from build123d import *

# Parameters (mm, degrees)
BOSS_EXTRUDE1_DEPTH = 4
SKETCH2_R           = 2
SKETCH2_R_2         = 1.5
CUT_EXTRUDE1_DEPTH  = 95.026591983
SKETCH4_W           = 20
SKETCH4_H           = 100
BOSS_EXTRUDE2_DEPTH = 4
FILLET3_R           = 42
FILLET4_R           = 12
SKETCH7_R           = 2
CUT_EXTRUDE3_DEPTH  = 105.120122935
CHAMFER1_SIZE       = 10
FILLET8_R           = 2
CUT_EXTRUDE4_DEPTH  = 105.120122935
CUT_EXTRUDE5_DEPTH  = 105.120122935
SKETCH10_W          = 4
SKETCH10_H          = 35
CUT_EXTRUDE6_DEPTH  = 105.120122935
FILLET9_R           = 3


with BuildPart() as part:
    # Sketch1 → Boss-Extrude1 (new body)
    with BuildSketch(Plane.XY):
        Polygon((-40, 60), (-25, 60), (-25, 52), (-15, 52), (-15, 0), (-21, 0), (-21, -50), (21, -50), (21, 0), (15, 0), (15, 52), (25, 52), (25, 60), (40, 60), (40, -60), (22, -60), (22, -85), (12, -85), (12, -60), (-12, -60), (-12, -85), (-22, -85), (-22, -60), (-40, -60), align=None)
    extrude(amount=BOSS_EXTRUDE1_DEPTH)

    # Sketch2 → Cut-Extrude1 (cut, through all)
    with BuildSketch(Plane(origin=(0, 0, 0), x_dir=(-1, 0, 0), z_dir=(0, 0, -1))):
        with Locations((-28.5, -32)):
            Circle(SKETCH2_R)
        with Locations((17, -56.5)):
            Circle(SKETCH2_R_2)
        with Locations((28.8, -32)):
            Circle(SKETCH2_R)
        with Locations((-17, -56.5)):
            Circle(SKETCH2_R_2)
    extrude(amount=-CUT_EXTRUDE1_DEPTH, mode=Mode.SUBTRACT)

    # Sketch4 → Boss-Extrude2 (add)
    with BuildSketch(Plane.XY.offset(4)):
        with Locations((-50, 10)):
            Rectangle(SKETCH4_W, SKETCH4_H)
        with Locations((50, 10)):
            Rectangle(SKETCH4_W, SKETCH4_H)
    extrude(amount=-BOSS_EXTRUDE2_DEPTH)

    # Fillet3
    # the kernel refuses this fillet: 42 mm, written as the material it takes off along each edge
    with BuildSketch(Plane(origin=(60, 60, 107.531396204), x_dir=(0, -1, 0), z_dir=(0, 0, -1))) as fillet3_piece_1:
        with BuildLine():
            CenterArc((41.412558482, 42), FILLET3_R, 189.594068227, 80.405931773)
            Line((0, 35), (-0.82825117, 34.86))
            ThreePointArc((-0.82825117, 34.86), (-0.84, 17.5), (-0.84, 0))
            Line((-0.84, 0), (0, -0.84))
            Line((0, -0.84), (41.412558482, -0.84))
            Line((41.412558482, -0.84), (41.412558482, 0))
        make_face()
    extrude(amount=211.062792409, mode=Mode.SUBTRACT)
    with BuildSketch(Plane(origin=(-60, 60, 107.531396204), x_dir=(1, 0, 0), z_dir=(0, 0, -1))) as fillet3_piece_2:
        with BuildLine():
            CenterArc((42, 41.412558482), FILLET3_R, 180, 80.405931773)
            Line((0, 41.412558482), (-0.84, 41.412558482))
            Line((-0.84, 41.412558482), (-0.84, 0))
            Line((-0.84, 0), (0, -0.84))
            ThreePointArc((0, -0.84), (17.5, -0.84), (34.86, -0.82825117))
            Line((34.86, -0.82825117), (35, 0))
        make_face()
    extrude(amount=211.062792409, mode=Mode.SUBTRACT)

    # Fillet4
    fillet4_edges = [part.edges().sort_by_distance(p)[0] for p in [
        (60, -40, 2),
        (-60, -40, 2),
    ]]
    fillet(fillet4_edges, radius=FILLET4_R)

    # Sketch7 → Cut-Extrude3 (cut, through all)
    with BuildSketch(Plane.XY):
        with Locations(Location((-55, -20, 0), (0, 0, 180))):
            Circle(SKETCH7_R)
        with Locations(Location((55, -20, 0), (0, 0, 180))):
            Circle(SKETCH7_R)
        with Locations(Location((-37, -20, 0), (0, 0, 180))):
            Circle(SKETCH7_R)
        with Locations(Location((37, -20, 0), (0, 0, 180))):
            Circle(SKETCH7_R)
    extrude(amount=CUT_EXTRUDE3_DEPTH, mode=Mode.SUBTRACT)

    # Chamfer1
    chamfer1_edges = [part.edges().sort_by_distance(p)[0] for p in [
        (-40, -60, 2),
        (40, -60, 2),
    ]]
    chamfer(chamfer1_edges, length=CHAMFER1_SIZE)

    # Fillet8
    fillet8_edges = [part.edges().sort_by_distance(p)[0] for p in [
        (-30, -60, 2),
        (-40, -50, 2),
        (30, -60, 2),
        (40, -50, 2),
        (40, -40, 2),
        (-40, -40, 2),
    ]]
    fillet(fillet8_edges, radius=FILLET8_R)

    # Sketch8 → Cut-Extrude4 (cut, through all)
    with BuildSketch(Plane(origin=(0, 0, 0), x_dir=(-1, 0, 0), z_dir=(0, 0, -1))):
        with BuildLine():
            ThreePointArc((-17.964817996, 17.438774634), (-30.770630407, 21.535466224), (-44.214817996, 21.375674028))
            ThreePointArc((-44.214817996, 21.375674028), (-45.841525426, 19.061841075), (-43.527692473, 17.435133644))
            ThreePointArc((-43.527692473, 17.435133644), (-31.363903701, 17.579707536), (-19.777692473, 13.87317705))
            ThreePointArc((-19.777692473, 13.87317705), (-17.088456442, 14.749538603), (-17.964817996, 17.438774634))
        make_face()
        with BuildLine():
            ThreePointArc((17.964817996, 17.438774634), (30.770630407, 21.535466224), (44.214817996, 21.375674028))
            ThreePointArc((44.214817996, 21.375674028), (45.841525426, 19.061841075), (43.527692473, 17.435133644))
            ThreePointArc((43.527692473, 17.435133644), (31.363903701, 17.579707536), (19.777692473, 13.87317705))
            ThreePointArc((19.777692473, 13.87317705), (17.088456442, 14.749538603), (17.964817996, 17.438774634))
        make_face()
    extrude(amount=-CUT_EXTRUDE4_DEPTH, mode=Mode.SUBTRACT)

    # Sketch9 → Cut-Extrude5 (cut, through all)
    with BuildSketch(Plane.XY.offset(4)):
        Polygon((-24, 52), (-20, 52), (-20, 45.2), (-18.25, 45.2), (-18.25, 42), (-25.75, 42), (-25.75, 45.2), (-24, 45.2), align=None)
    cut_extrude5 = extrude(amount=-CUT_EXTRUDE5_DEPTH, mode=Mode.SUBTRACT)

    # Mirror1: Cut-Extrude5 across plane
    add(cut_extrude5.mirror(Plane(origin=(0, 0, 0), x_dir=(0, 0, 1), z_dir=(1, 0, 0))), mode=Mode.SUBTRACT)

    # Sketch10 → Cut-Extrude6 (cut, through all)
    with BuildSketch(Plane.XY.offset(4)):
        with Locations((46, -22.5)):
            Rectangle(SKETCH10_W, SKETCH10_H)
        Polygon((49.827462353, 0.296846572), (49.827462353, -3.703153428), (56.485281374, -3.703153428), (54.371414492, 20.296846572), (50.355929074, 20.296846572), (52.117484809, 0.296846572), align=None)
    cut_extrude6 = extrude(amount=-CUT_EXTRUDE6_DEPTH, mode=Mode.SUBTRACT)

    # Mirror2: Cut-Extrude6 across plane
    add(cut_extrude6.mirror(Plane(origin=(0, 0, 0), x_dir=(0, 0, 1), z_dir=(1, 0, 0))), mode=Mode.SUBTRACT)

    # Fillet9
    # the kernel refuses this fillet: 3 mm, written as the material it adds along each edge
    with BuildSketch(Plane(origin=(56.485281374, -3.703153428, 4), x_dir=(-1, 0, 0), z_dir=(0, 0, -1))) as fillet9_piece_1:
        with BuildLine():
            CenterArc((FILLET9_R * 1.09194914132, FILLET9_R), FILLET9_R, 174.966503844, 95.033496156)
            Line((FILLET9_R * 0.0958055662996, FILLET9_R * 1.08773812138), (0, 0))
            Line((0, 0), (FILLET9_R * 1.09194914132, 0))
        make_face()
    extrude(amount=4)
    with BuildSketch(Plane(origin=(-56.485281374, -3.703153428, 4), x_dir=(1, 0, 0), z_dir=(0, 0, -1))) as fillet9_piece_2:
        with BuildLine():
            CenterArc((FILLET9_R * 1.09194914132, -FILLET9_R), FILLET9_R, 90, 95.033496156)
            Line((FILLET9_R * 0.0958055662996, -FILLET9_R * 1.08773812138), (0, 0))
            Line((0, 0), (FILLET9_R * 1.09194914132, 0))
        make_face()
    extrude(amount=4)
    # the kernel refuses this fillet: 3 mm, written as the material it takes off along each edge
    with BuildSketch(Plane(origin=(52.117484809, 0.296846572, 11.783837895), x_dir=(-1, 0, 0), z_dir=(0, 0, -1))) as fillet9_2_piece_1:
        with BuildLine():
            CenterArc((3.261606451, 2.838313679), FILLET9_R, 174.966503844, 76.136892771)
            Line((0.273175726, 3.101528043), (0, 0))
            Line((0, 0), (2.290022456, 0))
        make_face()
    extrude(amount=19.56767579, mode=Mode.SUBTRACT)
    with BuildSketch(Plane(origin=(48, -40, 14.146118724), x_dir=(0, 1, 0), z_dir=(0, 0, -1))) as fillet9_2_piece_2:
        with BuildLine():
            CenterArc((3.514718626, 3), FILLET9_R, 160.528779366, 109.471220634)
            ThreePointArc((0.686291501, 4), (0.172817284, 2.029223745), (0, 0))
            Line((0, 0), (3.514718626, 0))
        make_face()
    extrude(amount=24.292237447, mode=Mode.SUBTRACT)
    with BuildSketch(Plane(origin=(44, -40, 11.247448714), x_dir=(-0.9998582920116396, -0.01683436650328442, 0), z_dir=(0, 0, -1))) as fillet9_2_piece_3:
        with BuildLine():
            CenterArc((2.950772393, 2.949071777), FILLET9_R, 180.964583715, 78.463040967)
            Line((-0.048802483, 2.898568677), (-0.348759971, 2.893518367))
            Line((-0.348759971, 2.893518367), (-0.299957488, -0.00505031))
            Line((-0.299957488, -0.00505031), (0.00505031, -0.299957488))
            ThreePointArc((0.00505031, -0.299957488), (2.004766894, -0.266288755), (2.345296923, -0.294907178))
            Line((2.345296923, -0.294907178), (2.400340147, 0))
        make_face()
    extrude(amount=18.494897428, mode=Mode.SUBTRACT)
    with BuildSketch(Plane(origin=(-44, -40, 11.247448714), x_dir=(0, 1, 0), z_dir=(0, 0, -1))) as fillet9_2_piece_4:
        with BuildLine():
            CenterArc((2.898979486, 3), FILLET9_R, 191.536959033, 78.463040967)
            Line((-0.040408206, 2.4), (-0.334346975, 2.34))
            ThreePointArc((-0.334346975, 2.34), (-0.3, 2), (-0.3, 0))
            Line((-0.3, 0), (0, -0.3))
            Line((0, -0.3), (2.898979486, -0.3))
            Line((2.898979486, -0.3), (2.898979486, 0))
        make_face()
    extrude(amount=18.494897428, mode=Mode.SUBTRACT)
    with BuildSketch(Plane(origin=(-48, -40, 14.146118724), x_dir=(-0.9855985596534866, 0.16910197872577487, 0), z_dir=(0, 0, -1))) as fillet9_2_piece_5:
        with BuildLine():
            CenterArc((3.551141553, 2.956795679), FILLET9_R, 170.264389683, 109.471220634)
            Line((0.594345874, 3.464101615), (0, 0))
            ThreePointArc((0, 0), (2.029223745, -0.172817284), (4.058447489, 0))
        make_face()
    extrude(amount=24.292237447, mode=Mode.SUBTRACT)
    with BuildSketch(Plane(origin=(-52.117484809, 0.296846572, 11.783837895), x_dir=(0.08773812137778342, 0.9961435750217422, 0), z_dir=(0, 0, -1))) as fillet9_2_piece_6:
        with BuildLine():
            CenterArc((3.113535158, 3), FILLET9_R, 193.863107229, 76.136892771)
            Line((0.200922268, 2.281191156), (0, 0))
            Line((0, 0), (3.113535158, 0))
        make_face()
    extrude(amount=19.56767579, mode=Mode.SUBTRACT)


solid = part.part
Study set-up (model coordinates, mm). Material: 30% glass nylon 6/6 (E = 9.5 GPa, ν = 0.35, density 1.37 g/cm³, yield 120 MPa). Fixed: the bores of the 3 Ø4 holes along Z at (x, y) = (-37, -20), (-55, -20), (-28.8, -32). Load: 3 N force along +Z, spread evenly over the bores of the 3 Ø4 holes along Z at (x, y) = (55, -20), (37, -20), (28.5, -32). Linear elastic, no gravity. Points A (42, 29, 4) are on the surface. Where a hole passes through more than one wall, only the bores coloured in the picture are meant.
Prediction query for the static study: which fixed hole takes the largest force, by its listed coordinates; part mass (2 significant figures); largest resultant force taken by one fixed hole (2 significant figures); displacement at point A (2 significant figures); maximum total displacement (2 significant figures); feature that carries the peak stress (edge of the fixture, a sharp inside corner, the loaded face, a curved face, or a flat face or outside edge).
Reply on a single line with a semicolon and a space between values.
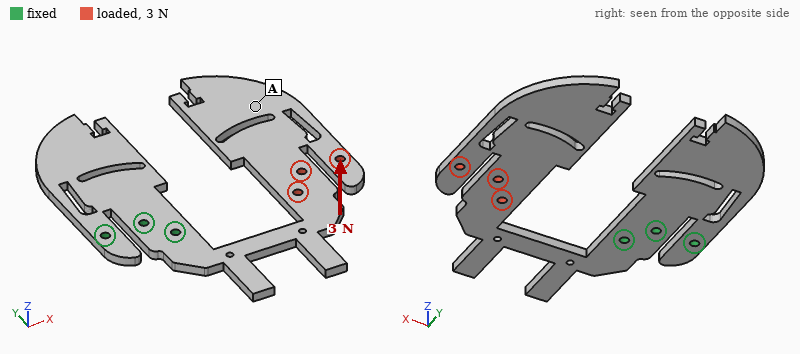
(-28.8, -32); 45 g; 3.7 N; 1.7 mm; 2.0 mm; a curved face
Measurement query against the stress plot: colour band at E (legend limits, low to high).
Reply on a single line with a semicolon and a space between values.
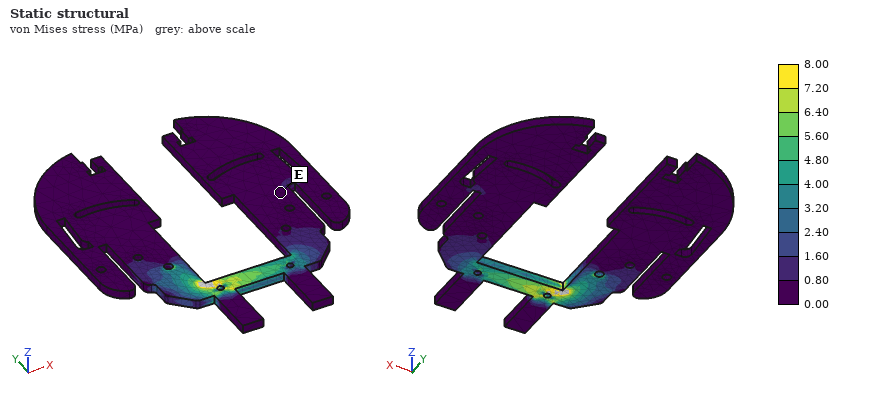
0.00 to 0.80 MPa
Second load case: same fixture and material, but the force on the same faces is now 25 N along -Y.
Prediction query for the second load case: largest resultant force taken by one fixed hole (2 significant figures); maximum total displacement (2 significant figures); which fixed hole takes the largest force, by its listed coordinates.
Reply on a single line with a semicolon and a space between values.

110 N; 2.1 mm; (-28.8, -32)
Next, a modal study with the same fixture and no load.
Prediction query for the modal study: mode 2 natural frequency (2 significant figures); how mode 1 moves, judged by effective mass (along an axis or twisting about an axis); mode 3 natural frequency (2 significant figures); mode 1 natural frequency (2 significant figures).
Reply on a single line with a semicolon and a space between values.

110 Hz; along Z; 130 Hz; 42 Hz
